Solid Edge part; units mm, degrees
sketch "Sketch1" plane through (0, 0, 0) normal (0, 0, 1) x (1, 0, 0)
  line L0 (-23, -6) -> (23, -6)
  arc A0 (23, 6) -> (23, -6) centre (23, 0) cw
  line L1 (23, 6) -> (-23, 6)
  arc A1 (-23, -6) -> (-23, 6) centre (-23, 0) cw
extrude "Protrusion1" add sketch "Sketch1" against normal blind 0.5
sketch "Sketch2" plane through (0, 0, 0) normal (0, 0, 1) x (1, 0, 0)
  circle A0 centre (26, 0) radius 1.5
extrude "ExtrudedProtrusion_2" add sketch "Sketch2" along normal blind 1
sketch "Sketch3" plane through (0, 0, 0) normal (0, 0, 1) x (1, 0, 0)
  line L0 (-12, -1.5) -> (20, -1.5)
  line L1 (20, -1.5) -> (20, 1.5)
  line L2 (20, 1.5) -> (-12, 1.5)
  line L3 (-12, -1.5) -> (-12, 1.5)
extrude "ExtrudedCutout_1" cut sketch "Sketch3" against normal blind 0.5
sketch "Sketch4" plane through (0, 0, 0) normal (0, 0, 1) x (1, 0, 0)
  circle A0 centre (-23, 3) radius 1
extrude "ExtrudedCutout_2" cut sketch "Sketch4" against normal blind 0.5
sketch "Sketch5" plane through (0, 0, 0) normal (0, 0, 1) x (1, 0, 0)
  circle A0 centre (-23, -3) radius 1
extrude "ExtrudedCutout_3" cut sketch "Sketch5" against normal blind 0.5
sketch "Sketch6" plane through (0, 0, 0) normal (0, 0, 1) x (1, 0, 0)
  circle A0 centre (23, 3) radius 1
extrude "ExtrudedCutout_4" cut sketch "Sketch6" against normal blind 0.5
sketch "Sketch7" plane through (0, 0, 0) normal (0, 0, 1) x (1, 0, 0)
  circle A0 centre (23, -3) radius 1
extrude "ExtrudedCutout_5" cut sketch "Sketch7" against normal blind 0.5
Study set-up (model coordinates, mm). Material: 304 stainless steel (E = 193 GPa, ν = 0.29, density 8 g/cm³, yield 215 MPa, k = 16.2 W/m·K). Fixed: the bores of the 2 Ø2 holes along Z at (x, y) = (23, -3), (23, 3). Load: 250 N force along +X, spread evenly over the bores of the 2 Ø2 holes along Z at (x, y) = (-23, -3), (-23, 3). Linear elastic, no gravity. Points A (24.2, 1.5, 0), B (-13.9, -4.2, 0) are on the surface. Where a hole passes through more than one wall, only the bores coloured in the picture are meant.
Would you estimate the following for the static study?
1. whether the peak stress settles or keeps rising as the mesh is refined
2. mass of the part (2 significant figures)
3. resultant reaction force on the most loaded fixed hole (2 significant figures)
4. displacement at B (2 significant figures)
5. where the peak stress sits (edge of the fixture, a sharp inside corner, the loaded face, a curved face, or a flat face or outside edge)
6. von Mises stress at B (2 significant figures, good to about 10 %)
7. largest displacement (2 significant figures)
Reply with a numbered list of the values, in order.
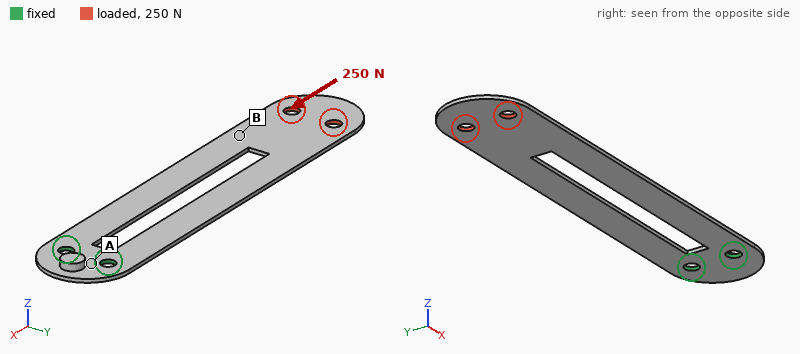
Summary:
1. keeps rising
2. 2.3 g
3. 130 N
4. 11 µm
5. edge of the fixture
6. 53 MPa
7. 13 µm
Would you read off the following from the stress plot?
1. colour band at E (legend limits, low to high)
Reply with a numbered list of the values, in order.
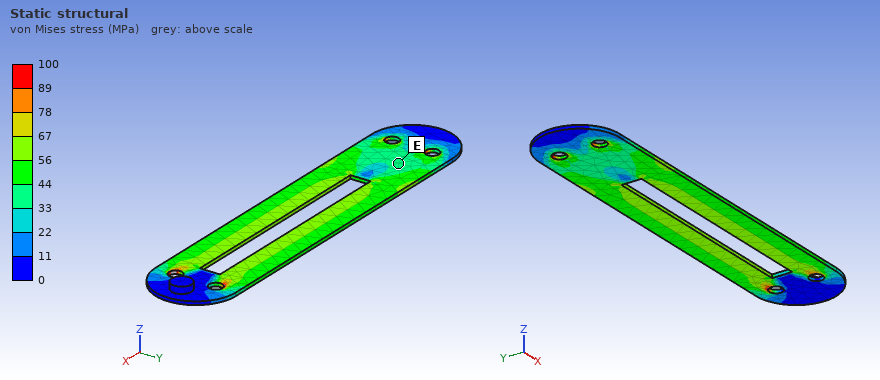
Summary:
1. 33 to 44 MPa
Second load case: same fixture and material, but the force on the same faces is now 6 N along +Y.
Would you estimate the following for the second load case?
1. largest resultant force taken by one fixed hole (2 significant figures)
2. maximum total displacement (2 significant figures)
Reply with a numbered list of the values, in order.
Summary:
1. 34 N
2. 34 µm
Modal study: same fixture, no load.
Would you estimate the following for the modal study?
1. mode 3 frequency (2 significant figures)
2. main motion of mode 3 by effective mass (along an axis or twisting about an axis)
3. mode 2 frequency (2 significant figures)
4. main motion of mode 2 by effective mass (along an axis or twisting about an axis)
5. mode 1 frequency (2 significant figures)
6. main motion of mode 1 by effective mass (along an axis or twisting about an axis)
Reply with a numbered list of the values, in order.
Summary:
1. 1100 Hz
2. twisting about X
3. 970 Hz
4. along Z
5. 150 Hz
6. along Z
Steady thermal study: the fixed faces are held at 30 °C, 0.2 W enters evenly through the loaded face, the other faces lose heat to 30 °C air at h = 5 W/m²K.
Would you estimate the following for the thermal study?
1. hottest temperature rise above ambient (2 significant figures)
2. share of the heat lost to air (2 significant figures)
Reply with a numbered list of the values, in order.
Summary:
1. 53 K
2. 71 %
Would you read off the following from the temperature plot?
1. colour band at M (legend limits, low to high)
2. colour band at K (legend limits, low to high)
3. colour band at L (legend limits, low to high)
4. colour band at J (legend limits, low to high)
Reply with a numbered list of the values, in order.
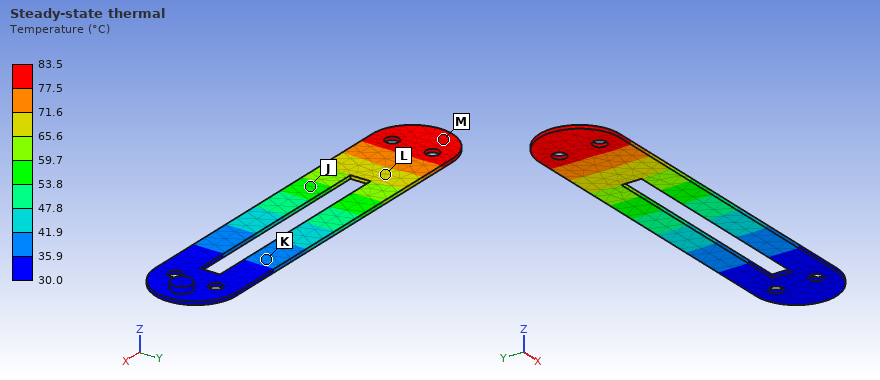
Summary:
1. 77.5 to 83.5 °C
2. 35.9 to 41.9 °C
3. 65.6 to 71.6 °C
4. 53.8 to 59.7 °C
